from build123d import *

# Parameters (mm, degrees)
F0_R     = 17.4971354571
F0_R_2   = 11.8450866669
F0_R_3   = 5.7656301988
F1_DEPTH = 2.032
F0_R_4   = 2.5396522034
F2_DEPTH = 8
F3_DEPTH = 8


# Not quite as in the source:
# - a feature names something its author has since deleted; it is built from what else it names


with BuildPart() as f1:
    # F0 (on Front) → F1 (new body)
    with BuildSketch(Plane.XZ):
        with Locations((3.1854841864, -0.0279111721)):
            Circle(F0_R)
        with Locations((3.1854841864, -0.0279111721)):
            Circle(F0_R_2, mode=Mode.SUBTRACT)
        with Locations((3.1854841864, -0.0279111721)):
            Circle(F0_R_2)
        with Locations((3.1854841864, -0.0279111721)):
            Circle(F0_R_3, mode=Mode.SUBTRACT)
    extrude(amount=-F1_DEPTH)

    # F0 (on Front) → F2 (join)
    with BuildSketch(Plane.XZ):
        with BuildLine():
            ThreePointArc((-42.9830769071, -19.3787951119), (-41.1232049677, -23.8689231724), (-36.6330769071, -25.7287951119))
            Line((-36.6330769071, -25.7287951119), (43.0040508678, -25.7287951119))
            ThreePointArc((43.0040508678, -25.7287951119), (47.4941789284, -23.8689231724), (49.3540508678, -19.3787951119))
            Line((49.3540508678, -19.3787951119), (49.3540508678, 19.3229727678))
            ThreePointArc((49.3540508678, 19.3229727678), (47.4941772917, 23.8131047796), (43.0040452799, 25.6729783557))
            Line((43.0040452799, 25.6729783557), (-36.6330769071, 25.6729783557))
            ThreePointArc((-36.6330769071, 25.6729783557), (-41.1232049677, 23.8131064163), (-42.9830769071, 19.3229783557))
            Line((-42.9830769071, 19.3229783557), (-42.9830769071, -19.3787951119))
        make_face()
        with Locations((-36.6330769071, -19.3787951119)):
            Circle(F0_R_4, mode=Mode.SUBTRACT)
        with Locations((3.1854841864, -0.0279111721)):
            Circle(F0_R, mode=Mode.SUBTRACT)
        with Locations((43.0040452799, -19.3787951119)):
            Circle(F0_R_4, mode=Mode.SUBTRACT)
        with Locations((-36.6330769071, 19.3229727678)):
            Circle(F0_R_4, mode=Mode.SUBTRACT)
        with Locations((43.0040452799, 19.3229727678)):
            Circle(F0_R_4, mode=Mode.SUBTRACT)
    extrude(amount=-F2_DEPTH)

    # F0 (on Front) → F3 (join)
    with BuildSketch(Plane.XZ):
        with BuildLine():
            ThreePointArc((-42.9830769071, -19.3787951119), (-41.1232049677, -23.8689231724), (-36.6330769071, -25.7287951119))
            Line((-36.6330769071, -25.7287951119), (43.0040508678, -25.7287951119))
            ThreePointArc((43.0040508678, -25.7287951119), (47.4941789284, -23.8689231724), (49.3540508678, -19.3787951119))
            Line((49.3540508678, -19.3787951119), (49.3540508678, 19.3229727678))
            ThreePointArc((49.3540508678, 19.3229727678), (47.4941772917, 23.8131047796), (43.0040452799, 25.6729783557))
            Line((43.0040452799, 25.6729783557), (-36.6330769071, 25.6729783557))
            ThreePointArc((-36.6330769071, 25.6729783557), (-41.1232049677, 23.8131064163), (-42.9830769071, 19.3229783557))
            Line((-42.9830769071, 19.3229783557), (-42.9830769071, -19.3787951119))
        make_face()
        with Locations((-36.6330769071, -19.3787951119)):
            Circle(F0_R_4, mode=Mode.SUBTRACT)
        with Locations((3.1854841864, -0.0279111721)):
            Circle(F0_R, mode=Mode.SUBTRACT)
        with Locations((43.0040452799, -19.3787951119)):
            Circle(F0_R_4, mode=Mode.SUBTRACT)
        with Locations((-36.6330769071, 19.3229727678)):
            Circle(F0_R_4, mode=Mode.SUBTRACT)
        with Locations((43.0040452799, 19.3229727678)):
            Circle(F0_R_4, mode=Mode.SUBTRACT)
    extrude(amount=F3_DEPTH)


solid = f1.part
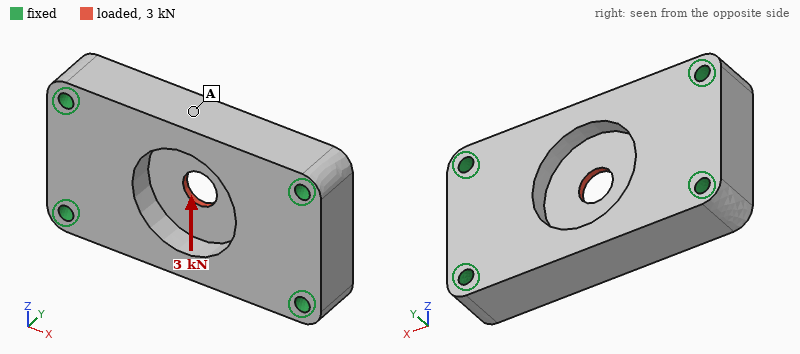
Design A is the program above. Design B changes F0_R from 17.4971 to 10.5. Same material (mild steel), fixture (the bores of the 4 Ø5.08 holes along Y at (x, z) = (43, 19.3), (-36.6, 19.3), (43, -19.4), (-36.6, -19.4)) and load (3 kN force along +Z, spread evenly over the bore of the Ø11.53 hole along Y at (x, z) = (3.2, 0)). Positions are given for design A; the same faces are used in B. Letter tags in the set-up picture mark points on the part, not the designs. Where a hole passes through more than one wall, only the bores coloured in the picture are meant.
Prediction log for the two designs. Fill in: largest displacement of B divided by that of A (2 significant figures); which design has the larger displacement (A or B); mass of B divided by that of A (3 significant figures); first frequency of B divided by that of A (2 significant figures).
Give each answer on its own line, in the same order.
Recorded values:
0.72
A
1.14
0.93
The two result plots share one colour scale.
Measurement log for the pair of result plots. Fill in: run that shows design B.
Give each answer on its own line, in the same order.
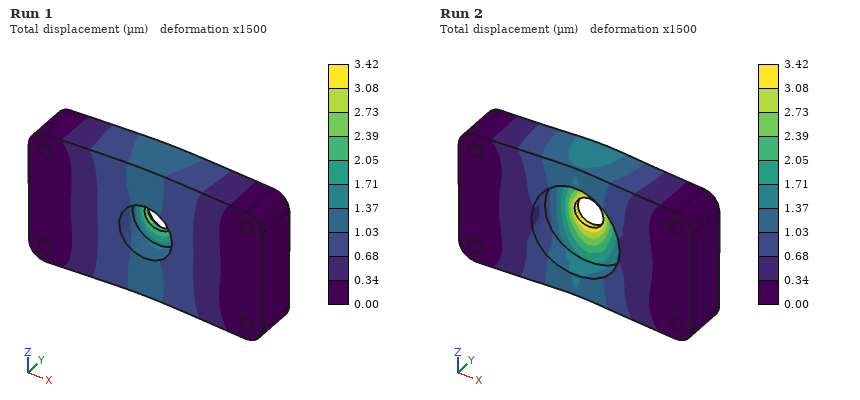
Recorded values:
Run 1
